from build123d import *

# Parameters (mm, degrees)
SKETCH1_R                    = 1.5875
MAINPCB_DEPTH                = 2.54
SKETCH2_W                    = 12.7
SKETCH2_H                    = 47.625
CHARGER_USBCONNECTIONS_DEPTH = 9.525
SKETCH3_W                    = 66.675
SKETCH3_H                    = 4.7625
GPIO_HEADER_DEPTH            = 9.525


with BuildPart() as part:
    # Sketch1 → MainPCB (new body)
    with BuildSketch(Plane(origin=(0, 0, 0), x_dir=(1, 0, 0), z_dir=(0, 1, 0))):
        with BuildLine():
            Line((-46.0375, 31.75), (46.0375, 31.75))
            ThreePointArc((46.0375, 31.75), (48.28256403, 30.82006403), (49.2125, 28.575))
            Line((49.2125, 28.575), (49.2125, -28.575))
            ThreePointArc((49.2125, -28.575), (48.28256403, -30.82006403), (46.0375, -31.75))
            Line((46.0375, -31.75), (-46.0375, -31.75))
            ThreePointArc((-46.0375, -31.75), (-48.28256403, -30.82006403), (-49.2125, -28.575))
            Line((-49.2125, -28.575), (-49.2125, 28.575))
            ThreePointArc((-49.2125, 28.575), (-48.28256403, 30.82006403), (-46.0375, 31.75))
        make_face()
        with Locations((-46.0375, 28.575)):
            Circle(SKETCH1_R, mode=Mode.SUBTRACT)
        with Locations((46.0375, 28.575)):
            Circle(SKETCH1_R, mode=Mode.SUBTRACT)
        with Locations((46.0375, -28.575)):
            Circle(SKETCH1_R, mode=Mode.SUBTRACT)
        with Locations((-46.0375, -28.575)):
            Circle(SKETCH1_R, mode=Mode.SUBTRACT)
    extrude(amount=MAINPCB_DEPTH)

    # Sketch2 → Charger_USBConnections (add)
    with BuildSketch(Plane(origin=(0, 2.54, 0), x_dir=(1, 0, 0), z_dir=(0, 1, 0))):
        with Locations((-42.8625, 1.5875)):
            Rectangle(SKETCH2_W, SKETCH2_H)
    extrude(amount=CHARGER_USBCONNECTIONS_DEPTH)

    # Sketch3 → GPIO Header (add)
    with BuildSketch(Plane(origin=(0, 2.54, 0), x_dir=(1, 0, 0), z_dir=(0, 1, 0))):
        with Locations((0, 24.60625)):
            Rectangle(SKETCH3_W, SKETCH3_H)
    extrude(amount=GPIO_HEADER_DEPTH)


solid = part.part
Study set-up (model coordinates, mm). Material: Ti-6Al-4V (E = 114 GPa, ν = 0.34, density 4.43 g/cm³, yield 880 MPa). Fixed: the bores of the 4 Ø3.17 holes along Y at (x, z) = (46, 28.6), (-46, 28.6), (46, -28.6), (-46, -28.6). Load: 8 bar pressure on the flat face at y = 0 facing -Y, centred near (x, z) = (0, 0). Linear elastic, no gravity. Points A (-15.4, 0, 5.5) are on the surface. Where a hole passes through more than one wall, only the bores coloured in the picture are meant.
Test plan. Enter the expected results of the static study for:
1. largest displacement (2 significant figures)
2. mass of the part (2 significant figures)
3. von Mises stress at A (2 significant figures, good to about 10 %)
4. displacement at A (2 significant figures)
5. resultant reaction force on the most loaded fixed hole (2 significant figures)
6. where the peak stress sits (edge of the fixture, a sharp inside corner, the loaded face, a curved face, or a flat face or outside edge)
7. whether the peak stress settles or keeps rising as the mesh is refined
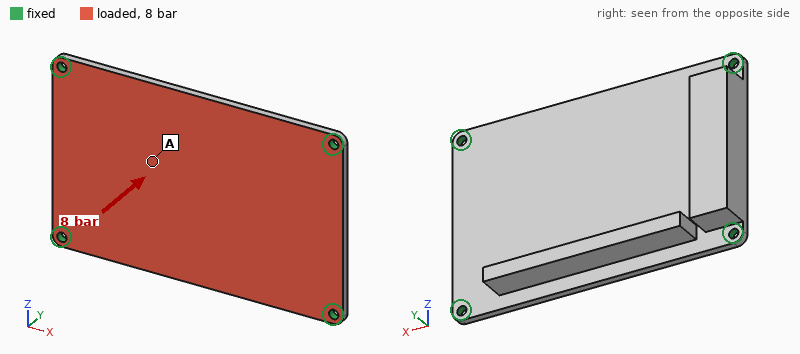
1.1 mm
110 g
150 MPa
0.64 mm
1.7 kN
edge of the fixture
keeps rising
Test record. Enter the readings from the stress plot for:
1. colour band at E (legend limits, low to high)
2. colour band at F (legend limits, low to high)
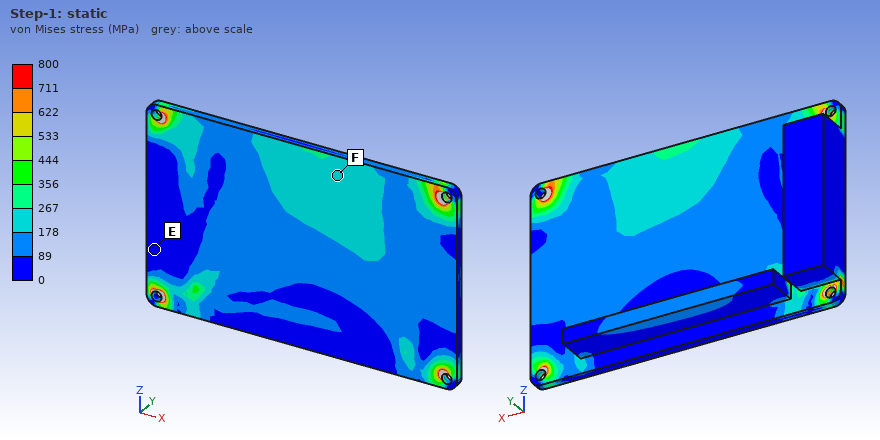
0 to 89 MPa
178 to 267 MPa
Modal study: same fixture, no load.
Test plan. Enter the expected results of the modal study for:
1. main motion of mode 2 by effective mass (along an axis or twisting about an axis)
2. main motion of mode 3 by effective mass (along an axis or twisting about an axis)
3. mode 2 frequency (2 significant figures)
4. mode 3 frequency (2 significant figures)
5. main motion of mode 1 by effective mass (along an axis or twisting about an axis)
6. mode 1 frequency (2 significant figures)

along Y
twisting about Z
3100 Hz
3600 Hz
along Y
1600 Hz
